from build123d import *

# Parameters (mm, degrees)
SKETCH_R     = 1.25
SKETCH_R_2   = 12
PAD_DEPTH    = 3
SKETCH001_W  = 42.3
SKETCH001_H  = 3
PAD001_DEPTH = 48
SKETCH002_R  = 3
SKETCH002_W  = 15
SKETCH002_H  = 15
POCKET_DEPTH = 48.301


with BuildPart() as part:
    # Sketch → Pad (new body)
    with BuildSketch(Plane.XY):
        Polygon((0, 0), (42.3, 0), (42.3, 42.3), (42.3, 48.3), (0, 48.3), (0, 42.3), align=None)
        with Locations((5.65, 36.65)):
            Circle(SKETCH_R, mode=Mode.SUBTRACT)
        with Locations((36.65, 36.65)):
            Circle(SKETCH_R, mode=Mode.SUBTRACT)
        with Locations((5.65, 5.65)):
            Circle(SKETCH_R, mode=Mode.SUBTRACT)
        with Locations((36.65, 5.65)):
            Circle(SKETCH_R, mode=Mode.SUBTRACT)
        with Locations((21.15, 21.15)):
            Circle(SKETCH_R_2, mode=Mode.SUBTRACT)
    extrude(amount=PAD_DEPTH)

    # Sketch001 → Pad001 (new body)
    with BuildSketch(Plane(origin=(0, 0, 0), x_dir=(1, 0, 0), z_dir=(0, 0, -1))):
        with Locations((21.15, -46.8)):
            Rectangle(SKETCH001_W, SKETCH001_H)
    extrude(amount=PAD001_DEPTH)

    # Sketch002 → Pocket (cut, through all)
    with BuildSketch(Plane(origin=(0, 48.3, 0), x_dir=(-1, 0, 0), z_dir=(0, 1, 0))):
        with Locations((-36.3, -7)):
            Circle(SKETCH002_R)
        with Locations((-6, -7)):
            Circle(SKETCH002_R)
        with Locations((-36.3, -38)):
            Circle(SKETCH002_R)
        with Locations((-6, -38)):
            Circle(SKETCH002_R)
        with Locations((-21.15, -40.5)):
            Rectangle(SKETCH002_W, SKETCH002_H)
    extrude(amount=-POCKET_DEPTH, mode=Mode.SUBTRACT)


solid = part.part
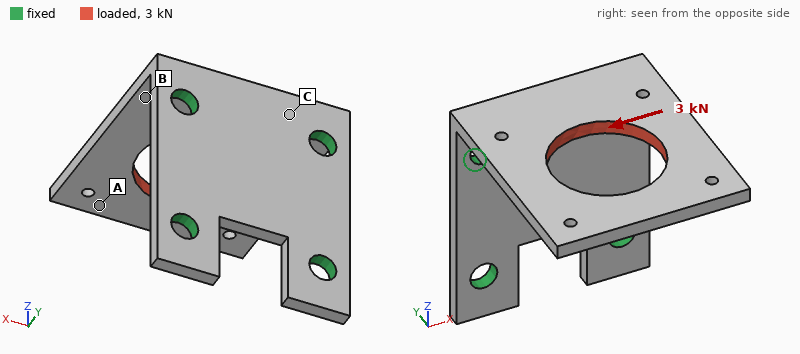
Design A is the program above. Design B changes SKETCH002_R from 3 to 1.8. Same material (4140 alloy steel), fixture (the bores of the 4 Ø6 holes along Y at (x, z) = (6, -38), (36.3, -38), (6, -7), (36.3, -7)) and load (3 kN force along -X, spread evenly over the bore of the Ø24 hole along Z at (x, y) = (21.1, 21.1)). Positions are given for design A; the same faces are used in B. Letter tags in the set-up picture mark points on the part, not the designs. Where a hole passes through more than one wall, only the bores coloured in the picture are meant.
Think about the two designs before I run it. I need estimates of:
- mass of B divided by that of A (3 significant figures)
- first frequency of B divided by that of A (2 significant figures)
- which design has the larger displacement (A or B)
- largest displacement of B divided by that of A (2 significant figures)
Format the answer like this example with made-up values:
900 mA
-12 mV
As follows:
1.02
0.96
B
1.4
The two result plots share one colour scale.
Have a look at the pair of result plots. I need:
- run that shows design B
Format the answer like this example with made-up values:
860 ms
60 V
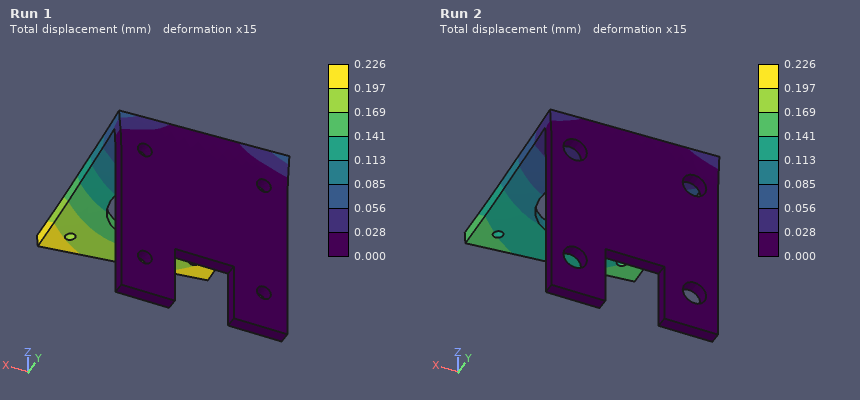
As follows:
Run 1
